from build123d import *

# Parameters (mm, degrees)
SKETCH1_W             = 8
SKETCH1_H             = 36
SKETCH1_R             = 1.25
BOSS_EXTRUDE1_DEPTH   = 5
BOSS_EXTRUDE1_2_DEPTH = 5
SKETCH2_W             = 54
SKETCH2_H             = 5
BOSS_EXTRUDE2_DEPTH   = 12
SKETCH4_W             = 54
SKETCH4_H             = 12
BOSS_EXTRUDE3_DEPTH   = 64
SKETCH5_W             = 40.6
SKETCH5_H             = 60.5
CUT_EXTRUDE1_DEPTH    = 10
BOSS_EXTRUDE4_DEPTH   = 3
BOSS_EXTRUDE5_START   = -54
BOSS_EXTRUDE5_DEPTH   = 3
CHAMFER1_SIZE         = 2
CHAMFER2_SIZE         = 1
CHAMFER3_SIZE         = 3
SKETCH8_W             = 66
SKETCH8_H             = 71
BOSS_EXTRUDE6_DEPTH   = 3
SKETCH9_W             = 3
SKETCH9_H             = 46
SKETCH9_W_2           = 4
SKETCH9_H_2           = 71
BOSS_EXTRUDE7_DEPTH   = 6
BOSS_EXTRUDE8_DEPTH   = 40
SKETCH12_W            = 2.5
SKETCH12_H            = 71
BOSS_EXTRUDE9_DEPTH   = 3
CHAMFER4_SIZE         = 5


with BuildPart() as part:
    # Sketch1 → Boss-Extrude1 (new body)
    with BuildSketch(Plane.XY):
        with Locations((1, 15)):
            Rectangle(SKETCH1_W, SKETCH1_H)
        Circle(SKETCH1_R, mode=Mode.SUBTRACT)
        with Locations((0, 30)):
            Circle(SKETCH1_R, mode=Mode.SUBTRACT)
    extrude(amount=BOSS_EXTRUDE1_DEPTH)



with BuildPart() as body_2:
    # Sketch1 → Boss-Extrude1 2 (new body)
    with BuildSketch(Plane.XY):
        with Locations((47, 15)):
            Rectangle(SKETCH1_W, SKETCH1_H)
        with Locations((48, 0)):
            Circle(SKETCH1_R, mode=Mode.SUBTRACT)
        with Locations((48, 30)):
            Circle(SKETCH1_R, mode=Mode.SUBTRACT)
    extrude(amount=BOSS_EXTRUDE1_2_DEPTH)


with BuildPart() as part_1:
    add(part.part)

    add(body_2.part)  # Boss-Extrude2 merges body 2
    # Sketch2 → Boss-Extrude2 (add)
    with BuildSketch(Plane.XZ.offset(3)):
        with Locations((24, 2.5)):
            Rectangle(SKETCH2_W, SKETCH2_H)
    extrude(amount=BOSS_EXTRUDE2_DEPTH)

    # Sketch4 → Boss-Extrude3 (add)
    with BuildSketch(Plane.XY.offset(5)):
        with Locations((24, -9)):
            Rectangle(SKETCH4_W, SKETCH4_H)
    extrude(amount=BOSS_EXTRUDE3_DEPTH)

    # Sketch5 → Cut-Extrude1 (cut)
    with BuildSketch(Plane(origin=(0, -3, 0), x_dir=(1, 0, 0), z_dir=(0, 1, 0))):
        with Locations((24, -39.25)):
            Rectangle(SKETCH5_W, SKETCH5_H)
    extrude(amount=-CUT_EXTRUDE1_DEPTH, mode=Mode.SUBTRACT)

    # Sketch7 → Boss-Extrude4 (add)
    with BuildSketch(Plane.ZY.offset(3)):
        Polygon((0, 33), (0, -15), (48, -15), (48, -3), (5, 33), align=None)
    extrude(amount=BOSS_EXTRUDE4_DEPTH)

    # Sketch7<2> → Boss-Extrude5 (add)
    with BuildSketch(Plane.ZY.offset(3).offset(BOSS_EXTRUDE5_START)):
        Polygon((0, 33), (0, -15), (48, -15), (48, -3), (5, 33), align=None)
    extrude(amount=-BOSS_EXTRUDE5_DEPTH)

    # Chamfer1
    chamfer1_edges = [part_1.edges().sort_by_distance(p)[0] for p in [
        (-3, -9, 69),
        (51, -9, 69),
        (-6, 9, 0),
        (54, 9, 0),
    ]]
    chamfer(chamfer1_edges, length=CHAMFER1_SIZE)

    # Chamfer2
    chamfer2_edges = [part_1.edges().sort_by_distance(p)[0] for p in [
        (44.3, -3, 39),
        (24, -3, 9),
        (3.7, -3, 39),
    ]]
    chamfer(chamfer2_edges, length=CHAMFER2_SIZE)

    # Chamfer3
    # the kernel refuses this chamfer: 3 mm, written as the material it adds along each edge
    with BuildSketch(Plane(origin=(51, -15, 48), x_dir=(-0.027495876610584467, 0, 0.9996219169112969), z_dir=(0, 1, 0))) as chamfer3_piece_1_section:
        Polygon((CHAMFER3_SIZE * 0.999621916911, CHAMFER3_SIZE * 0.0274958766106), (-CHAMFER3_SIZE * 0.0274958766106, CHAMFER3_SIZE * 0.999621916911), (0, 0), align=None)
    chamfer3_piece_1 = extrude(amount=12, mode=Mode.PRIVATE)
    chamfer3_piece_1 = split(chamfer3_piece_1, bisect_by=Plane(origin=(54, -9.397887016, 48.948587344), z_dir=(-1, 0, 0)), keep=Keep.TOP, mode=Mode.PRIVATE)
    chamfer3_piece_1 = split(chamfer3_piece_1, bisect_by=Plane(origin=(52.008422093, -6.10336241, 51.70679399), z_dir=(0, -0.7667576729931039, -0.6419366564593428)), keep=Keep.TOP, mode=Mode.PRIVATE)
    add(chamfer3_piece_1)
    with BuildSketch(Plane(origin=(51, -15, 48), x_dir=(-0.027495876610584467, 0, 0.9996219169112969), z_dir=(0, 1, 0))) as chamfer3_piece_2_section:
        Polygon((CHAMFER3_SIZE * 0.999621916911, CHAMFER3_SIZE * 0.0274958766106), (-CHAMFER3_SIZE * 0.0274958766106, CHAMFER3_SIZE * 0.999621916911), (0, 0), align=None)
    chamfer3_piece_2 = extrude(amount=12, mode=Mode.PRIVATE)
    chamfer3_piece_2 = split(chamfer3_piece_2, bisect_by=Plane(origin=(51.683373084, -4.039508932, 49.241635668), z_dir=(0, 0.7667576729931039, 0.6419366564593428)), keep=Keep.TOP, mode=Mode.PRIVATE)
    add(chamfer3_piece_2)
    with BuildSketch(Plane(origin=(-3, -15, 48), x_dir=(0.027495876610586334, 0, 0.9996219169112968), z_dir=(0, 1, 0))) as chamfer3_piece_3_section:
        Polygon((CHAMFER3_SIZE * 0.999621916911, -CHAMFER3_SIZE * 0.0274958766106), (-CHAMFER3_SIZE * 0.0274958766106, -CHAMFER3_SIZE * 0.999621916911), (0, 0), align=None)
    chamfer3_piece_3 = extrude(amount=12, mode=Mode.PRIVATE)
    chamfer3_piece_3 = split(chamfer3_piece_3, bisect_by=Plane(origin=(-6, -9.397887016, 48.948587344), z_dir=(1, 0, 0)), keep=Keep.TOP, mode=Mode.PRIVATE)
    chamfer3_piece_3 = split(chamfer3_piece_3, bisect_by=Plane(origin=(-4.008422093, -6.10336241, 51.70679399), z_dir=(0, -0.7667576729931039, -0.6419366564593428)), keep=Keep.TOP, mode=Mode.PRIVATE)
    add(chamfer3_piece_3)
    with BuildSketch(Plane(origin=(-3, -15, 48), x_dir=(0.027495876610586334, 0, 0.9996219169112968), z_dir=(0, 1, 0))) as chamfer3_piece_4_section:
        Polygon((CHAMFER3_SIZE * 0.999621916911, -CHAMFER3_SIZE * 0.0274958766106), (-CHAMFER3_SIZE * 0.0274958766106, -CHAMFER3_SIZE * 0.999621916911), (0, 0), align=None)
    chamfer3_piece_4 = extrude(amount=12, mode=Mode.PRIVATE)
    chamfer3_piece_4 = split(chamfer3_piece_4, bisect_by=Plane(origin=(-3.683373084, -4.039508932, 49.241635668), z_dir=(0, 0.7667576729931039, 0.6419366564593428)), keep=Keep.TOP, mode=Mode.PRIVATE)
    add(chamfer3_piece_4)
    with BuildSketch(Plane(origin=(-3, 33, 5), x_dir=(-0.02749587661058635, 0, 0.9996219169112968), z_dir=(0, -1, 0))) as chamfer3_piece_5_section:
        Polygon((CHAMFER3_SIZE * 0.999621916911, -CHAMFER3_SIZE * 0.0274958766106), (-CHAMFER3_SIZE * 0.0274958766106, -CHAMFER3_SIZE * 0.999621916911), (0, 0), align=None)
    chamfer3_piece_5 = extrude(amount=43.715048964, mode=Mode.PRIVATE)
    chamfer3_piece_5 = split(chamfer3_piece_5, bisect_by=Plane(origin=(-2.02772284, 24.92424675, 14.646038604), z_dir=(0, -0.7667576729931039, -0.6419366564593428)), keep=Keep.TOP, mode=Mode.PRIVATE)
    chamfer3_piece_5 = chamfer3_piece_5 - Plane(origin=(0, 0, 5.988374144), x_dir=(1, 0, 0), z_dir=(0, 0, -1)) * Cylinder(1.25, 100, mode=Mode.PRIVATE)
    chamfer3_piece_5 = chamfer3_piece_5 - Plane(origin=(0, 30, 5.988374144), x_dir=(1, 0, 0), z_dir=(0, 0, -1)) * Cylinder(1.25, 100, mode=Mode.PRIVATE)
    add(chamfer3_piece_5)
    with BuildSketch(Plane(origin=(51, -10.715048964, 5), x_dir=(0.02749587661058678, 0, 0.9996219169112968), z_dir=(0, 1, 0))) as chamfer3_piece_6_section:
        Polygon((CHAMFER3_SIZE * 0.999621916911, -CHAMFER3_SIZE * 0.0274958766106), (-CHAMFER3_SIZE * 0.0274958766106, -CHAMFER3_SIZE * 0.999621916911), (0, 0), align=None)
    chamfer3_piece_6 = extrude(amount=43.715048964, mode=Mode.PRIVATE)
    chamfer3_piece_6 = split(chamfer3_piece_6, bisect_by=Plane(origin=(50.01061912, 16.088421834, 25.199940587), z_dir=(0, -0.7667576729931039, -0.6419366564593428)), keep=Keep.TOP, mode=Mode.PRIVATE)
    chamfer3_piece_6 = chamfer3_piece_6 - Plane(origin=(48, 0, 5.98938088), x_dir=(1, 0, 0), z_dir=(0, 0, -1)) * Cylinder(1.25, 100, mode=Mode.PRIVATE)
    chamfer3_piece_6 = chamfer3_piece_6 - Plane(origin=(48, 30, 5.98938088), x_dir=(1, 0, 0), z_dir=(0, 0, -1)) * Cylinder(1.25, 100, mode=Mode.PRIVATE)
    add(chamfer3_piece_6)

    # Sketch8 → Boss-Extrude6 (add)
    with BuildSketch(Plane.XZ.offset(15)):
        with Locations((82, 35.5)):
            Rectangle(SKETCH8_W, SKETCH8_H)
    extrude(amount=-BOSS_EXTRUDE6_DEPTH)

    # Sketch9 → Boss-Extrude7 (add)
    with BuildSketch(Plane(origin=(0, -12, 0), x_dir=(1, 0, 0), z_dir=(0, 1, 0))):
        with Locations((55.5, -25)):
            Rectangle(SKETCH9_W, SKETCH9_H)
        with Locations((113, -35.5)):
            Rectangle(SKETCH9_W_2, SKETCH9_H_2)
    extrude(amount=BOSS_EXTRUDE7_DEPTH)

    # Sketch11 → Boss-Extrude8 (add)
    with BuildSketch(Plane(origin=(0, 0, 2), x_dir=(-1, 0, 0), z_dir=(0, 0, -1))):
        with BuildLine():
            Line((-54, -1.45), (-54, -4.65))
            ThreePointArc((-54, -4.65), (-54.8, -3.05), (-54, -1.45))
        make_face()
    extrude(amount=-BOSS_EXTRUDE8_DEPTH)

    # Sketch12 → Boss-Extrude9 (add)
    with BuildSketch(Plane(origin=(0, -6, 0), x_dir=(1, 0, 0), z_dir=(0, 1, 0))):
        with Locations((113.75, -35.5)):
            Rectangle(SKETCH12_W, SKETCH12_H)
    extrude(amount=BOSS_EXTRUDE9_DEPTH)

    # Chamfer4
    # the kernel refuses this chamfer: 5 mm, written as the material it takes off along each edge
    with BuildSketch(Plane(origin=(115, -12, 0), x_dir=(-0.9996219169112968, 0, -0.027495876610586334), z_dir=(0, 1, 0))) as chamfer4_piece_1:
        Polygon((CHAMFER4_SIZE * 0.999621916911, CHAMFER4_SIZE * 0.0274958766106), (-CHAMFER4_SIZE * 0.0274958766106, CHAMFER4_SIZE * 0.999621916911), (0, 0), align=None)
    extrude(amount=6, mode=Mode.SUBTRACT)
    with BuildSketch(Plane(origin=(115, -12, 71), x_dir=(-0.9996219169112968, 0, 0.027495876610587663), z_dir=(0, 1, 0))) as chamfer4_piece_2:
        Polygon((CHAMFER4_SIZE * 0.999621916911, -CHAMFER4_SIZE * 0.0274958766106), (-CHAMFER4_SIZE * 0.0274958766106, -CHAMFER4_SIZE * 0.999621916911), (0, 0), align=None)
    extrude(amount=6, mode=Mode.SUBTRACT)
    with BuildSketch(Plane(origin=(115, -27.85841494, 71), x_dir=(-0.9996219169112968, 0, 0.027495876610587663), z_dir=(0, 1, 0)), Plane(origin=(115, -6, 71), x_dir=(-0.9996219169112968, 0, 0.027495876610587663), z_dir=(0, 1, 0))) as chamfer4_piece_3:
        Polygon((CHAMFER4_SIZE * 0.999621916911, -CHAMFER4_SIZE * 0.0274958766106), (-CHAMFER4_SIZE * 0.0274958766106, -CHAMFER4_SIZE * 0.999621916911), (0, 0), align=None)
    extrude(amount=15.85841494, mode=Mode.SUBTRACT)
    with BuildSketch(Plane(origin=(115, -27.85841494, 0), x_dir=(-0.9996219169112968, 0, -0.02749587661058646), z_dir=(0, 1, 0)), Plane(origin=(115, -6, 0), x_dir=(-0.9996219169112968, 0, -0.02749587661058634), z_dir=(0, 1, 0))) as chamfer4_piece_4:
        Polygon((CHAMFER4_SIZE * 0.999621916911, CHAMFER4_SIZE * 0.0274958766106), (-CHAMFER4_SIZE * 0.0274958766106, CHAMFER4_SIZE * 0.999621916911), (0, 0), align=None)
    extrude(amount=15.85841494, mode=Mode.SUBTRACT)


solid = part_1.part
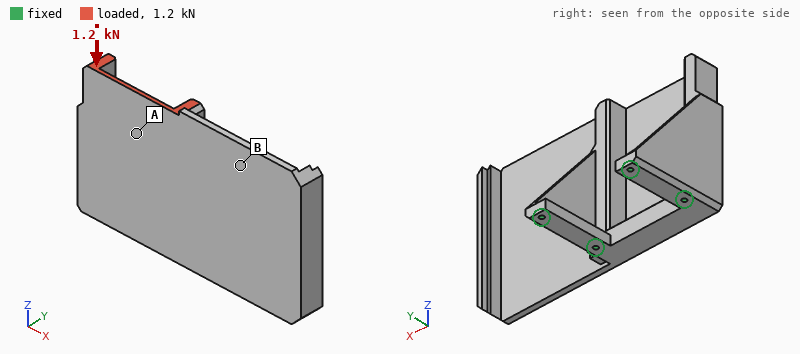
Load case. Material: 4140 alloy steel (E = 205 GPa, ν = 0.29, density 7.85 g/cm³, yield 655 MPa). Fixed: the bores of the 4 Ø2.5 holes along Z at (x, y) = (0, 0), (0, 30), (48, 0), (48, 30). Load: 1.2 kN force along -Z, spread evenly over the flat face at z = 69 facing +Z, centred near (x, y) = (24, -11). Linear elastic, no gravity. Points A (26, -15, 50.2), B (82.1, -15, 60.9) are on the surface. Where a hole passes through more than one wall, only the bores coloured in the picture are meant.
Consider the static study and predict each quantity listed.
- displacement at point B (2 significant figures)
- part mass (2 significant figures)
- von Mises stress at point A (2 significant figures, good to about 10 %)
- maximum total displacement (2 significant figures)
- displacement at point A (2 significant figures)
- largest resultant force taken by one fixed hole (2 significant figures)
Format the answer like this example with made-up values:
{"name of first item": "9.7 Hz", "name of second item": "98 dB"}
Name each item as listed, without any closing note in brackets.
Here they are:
{"displacement at point B": "5.3 µm", "part mass": "380 g", "von Mises stress at point A": "5.5 MPa", "maximum total displacement": "11 µm", "displacement at point A": "7.8 µm", "largest resultant force taken by one fixed hole": "800 N"}
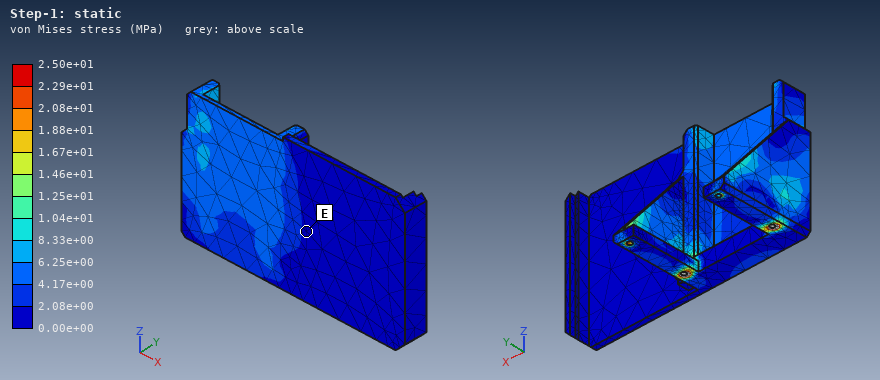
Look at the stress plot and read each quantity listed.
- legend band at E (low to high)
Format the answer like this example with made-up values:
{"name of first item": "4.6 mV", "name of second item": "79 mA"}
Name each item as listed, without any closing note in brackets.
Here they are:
{"legend band at E": "0.00e+00 to 2.08e+00 MPa"}
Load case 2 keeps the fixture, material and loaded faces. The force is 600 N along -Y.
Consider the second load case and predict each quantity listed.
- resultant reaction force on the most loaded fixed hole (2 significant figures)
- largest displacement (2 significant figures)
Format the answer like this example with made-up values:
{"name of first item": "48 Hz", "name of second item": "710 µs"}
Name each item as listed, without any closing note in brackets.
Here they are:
{"resultant reaction force on the most loaded fixed hole": "740 N", "largest displacement": "85 µm"}
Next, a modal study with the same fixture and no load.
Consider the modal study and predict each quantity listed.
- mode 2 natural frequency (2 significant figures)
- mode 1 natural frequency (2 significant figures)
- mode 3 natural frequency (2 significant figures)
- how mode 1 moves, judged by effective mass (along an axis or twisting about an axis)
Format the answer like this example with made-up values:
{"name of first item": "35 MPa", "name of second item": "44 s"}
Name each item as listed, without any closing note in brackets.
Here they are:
{"mode 2 natural frequency": "1300 Hz", "mode 1 natural frequency": "510 Hz", "mode 3 natural frequency": "2000 Hz", "how mode 1 moves, judged by effective mass": "along Y"}
